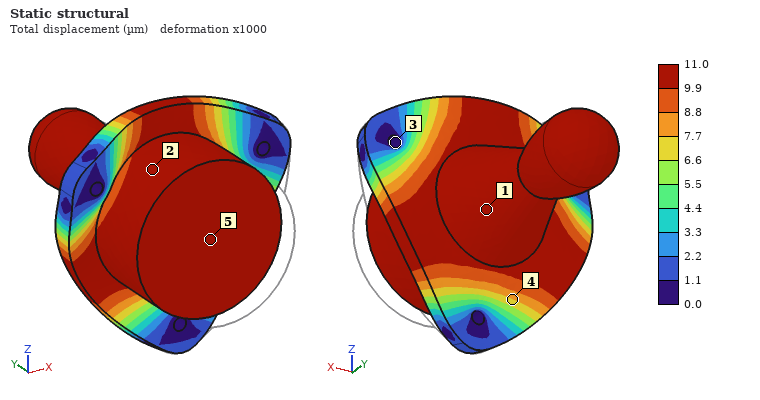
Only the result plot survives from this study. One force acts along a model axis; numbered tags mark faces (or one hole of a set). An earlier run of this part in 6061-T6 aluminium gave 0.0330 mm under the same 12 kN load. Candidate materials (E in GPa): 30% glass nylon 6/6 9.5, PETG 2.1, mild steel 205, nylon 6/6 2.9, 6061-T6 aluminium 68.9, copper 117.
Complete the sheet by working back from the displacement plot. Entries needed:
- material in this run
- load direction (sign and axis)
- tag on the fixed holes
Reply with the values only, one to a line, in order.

mild steel
+Y
3
